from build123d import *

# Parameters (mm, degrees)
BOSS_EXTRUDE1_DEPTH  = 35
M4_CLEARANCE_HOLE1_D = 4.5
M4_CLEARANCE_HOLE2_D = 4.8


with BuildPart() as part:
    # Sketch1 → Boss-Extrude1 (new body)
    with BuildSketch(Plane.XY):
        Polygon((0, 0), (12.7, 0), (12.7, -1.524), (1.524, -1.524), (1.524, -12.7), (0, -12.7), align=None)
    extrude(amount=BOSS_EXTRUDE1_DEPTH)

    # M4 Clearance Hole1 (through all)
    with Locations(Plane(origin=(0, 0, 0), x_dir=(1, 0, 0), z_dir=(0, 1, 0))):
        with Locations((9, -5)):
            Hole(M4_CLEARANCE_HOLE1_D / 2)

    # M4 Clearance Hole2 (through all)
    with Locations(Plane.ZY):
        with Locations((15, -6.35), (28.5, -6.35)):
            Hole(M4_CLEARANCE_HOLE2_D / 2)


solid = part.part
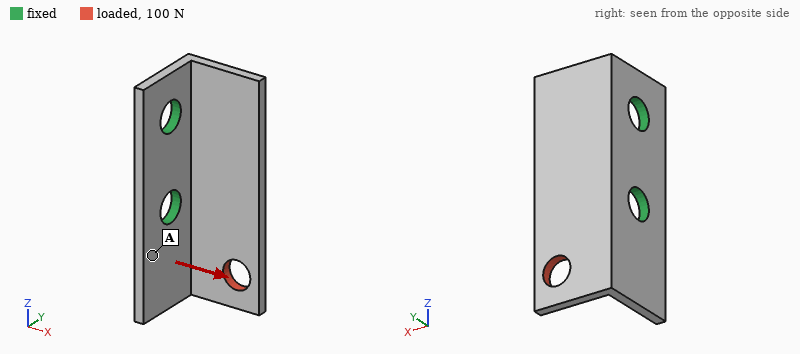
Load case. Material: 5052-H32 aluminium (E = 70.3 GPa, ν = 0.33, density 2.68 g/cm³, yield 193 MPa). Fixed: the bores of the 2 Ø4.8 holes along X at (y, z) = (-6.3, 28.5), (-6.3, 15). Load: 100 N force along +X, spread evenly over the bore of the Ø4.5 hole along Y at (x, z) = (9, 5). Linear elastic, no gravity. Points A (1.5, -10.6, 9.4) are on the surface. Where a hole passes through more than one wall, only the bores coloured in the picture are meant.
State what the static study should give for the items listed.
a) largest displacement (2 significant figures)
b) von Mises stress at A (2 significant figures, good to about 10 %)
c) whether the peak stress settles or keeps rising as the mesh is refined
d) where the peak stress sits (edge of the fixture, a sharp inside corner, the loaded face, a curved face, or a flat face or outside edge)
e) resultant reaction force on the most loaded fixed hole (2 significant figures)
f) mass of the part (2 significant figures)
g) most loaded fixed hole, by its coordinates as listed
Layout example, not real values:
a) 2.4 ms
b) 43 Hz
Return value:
a) 52 µm
b) 17 MPa
c) keeps rising
d) edge of the fixture
e) 150 N
f) 3.2 g
g) (-6.3, 15)
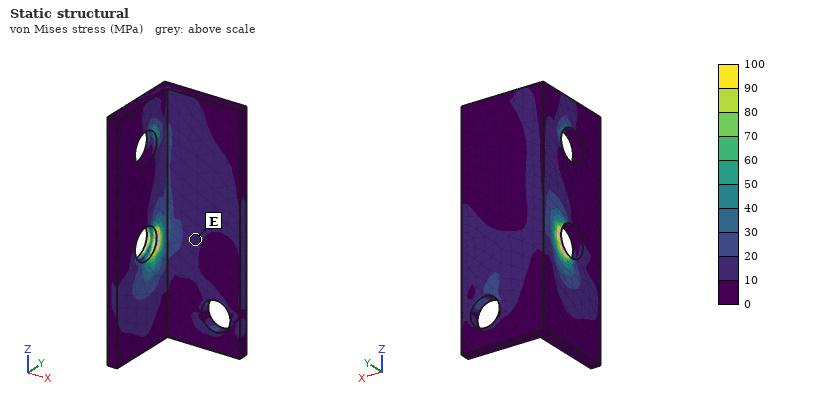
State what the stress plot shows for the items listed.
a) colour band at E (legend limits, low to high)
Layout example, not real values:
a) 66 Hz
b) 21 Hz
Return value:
a) 10 to 20 MPa
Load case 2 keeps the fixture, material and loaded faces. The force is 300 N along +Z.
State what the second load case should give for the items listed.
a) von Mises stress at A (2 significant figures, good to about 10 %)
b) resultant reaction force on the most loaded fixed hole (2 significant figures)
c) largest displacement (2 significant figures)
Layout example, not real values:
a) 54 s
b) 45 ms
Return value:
a) 18 MPa
b) 230 N
c) 59 µm
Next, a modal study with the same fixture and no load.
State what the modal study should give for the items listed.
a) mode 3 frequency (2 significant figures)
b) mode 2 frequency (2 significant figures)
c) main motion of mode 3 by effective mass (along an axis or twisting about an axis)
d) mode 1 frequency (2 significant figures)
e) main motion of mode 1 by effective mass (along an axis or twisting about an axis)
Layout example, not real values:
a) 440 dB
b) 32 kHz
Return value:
a) 11 kHz
b) 8100 Hz
c) along X
d) 5800 Hz
e) along Y
